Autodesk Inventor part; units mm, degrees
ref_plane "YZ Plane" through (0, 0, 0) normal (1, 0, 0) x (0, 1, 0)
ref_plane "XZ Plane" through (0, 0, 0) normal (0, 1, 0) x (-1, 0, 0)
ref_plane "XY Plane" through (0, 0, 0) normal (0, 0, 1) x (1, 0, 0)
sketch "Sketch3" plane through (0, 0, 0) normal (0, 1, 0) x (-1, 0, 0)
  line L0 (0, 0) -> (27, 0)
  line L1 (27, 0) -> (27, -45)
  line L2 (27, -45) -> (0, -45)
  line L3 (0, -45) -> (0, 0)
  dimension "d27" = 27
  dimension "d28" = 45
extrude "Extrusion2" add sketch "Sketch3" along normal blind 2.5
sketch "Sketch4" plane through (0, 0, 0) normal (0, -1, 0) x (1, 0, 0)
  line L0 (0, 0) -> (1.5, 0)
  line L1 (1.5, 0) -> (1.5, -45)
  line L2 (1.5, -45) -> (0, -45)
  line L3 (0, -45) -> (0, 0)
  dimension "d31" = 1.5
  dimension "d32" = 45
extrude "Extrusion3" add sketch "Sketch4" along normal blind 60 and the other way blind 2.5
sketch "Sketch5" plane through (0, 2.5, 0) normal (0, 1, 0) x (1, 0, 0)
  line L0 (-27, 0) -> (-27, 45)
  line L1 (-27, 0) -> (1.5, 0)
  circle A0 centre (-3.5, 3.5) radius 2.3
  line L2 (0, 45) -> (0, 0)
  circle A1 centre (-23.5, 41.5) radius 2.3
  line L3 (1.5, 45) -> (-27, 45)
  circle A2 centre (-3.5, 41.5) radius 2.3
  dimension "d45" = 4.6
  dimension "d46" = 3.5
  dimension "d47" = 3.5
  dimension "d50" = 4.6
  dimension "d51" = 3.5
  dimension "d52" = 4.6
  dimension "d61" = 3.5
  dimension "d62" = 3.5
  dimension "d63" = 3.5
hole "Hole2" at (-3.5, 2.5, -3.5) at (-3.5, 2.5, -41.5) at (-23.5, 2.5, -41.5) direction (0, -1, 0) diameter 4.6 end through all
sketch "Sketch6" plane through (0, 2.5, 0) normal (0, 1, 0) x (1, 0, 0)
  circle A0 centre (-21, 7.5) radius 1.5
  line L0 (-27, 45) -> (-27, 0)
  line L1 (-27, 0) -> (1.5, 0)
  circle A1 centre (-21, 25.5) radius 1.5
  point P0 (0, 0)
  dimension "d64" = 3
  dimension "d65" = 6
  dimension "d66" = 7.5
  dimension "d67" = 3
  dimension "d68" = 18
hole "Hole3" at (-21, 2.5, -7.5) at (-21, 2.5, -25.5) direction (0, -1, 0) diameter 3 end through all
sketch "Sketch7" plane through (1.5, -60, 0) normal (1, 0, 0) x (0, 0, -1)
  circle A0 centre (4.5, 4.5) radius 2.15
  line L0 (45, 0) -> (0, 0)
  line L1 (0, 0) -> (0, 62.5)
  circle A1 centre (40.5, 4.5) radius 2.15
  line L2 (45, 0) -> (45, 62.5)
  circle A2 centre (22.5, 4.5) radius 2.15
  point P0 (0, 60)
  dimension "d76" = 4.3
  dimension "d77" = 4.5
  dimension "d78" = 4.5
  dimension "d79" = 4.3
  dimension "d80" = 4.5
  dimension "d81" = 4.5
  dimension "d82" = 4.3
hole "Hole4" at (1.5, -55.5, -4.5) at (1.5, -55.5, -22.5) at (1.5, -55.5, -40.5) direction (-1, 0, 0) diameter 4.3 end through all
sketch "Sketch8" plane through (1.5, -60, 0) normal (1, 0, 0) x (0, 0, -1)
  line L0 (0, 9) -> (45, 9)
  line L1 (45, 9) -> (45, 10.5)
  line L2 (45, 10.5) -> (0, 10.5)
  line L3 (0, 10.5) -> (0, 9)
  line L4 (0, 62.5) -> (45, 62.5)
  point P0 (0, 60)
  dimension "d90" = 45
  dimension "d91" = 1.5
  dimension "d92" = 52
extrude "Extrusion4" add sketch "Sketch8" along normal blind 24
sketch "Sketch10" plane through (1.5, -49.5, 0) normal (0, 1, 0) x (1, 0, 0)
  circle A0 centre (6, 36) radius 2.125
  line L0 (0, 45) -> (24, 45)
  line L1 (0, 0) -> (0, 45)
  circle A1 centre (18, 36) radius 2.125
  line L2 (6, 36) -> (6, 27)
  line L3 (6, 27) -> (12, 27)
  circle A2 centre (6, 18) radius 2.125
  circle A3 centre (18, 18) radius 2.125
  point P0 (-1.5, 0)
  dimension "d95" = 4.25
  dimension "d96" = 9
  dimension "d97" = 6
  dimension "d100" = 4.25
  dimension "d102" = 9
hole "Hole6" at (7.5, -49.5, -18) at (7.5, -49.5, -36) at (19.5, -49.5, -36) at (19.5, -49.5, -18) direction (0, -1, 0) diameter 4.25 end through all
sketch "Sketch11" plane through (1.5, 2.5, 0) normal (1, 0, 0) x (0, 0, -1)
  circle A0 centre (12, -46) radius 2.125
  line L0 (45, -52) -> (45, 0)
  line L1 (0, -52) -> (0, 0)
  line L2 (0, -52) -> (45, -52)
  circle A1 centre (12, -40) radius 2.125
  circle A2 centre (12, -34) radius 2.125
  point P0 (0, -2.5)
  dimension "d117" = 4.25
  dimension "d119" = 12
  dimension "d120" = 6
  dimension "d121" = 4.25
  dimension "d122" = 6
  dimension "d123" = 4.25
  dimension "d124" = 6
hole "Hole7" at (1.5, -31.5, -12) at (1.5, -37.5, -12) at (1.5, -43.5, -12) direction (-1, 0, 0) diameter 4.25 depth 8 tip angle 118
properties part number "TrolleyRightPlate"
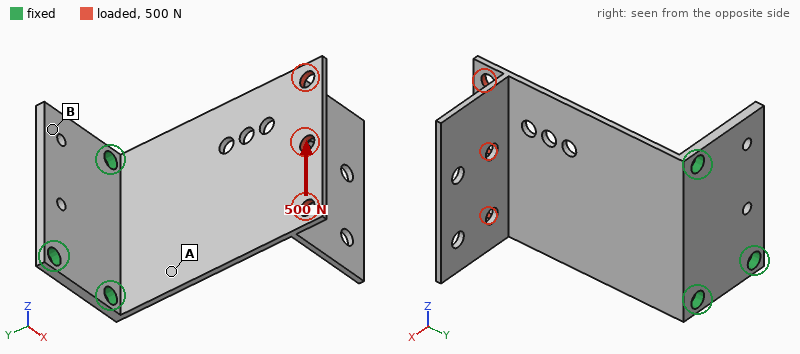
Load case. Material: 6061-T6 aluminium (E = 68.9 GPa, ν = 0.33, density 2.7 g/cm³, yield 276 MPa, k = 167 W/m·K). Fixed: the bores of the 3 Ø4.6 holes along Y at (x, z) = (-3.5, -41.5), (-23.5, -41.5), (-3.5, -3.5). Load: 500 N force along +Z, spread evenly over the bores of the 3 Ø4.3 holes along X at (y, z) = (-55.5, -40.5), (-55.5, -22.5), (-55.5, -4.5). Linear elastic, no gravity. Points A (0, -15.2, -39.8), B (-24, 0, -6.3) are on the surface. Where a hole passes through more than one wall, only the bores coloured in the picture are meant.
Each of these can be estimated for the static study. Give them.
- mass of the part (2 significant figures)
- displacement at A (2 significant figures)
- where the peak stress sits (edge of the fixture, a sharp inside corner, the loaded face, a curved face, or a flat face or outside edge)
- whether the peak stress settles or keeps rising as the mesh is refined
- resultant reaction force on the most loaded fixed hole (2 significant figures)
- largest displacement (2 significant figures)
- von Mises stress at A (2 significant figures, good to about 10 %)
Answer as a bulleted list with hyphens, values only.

- 23 g
- 0.037 mm
- edge of the fixture
- keeps rising
- 800 N
- 0.12 mm
- 37 MPa
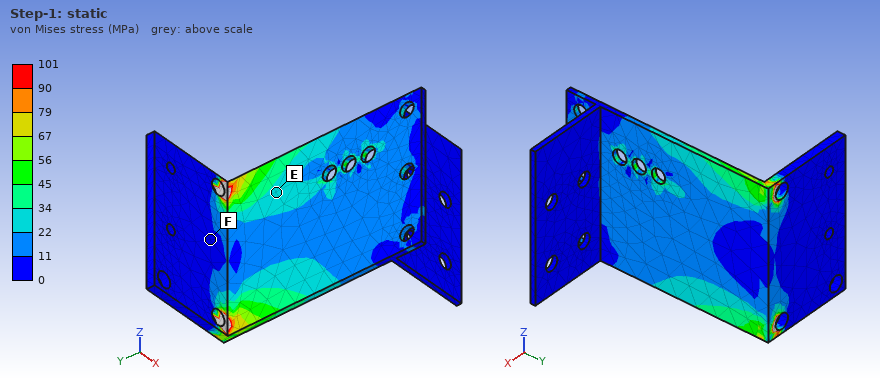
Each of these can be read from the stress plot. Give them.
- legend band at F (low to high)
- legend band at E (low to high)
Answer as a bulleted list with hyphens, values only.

- 0 to 11 MPa
- 22 to 34 MPa
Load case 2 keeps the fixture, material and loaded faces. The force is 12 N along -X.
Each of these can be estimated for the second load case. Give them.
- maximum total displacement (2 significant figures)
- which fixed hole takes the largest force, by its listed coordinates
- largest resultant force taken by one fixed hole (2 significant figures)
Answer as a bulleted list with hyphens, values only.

- 0.90 mm
- (-3.5, -41.5)
- 11 N
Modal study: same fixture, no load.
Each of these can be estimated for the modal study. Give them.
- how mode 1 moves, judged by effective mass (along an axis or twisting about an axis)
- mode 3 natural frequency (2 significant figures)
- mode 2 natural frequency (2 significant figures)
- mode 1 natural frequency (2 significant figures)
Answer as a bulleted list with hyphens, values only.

- along X
- 1100 Hz
- 630 Hz
- 240 Hz
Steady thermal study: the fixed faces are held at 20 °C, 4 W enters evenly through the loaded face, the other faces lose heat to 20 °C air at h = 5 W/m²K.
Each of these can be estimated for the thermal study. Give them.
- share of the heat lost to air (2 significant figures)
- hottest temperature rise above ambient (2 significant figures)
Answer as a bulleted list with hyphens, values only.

- 13 %
- 22 K
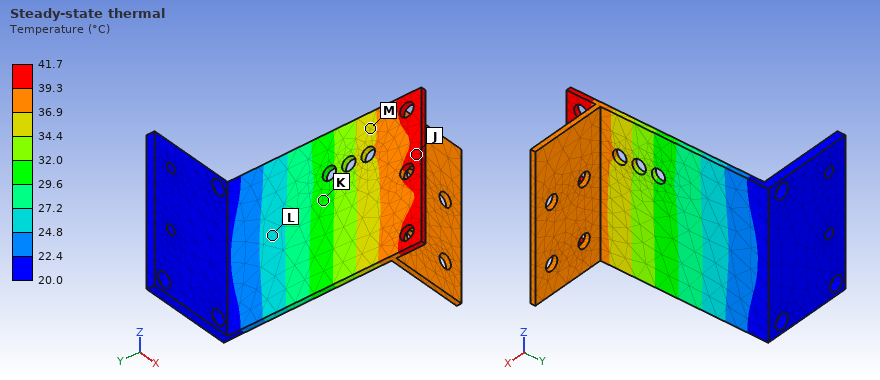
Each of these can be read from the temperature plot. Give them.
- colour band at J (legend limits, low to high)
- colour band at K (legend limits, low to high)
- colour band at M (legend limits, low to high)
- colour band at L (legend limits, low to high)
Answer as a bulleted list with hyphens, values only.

- 39.3 to 41.7 °C
- 29.6 to 32.0 °C
- 34.4 to 36.9 °C
- 24.8 to 27.2 °C
